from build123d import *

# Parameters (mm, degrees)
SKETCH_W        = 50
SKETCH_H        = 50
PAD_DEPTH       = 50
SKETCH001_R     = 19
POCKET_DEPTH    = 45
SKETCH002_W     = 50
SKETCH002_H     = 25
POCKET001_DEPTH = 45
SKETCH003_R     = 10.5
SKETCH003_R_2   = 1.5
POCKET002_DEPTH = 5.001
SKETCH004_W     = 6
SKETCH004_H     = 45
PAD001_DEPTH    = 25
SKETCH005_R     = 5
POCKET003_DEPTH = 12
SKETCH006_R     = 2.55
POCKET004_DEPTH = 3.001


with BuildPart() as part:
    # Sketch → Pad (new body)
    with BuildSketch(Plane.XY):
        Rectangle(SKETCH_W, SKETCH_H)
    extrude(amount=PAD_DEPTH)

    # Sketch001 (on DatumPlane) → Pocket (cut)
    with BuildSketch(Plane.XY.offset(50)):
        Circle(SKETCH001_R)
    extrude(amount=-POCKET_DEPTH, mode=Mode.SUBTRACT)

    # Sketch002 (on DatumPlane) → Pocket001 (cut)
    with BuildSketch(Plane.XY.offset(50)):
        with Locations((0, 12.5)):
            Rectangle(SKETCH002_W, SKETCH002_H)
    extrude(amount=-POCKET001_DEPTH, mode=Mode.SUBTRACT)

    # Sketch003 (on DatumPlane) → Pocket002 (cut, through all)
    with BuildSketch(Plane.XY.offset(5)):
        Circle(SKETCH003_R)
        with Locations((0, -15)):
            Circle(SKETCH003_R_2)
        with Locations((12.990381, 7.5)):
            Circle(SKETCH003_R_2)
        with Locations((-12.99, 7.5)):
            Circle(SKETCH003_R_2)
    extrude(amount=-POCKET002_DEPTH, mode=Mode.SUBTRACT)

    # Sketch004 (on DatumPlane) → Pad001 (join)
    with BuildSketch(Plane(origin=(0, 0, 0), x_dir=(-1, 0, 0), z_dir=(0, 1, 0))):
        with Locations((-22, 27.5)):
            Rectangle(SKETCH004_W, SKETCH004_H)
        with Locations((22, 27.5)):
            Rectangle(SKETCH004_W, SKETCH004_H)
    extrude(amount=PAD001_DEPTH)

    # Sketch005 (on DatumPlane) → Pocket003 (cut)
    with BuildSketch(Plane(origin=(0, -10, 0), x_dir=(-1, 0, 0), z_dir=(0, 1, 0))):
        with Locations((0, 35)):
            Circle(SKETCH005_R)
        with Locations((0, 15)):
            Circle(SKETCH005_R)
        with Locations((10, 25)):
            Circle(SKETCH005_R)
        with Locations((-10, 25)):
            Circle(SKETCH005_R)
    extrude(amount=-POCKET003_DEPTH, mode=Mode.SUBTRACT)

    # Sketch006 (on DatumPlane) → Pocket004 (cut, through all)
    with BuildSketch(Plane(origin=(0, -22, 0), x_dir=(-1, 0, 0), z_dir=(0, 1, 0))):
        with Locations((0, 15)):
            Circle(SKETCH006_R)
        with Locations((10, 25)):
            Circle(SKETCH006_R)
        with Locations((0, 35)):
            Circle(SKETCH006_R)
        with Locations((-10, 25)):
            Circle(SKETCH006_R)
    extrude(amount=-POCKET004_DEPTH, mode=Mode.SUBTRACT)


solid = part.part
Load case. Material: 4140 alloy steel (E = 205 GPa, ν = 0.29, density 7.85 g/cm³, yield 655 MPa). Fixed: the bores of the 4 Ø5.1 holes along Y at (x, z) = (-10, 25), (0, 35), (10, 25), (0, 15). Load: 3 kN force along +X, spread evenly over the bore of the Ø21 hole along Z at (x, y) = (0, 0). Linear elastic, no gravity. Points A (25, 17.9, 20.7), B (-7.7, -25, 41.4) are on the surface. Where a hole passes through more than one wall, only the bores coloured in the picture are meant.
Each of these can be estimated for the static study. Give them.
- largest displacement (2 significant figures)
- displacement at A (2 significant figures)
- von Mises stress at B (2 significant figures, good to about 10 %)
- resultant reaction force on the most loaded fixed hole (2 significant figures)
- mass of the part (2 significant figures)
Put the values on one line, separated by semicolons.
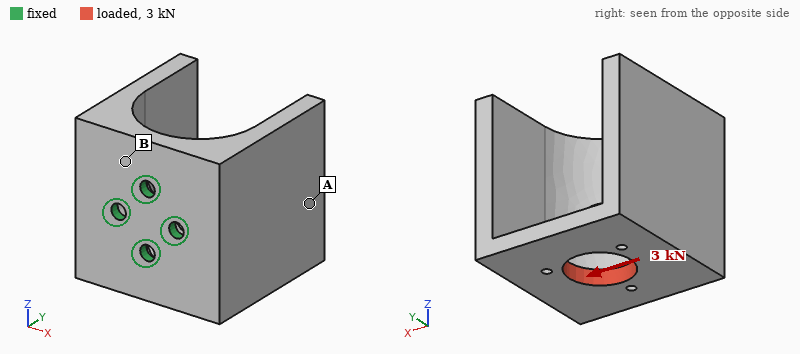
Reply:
61 µm; 47 µm; 35 MPa; 3.2 kN; 420 g
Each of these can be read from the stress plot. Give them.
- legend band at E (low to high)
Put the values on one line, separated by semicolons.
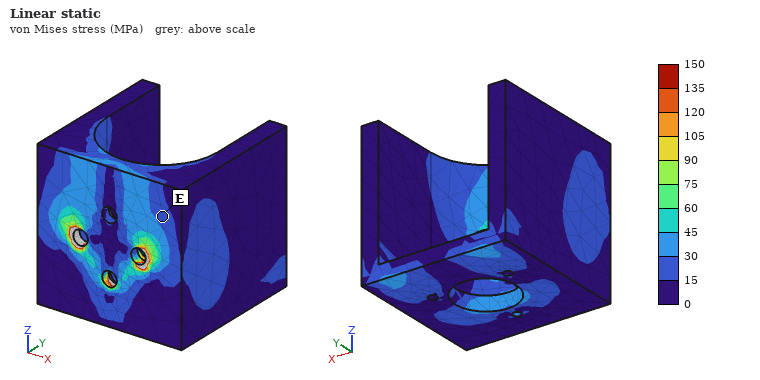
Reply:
15 to 30 MPa
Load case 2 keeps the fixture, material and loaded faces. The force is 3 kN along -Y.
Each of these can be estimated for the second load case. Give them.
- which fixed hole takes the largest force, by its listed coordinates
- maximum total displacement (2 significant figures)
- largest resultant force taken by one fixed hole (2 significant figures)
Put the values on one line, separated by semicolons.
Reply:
(0, 15); 37 µm; 3.3 kN
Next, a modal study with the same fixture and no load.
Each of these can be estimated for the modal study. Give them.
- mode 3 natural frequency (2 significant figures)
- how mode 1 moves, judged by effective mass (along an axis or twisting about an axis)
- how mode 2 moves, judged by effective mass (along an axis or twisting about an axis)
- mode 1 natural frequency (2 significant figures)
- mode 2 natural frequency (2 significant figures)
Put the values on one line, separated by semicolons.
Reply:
4200 Hz; along X; along Z; 2400 Hz; 2600 Hz
